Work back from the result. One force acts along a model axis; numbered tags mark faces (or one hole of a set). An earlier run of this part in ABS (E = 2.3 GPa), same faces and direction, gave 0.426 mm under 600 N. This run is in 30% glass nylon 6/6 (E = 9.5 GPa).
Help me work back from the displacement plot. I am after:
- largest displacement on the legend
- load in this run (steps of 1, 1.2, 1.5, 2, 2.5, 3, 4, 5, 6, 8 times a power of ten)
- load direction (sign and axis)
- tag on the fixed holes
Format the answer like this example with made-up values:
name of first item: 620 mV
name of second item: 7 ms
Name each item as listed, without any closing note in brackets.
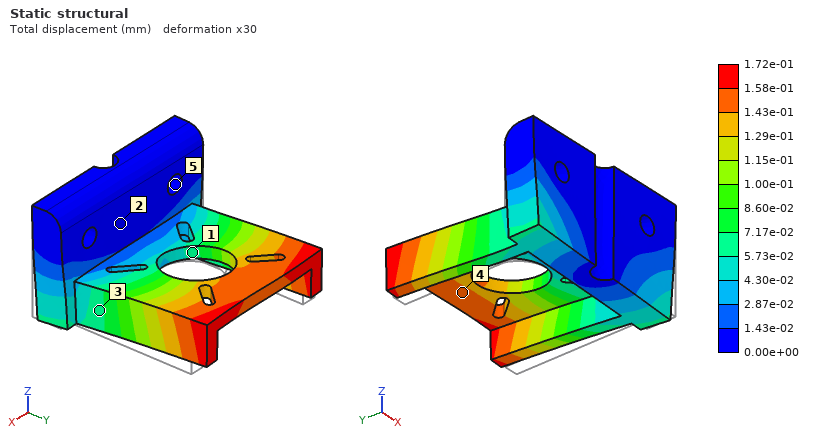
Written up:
largest displacement on the legend: 1.72e-01 mm
load in this run: 1 kN
load direction: -X
tag on the fixed holes: 5
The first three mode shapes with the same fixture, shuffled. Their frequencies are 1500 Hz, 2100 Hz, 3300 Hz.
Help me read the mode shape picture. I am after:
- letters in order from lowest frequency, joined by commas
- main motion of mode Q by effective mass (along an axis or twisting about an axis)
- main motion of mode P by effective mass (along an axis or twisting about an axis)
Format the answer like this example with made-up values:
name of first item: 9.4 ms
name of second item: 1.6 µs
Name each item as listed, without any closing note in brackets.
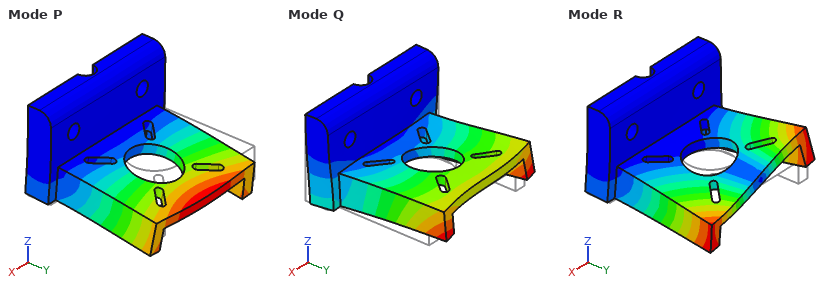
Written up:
letters in order from lowest frequency, joined by commas: P, R, Q
main motion of mode Q by effective mass: along X
main motion of mode P by effective mass: along Z
